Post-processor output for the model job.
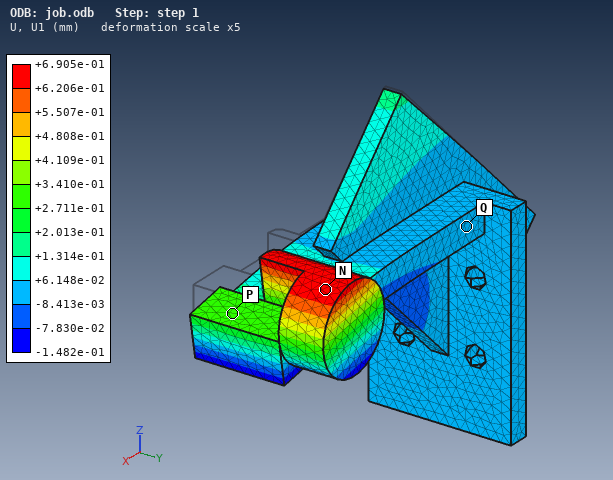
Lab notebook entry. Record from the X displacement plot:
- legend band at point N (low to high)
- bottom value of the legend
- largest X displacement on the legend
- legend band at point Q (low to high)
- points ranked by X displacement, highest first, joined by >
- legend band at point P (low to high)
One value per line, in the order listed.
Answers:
+6.206e-01 to +6.905e-01 mm
-1.482e-01 mm
+6.905e-01 mm
-8.413e-03 to +6.148e-02 mm
N > P > Q
+2.711e-01 to +3.410e-01 mm
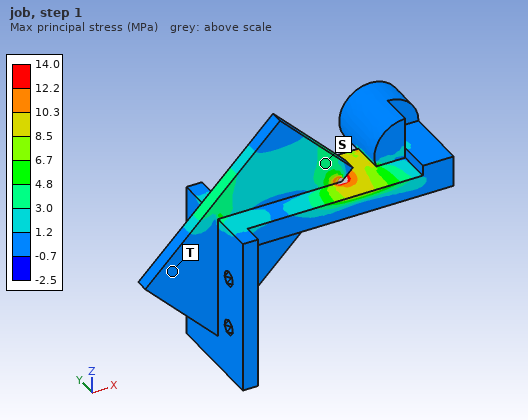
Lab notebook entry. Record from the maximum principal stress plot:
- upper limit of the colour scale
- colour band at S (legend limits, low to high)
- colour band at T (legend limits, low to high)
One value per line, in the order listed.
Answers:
14.0 MPa
3.0 to 4.8 MPa
-0.7 to 1.2 MPa
